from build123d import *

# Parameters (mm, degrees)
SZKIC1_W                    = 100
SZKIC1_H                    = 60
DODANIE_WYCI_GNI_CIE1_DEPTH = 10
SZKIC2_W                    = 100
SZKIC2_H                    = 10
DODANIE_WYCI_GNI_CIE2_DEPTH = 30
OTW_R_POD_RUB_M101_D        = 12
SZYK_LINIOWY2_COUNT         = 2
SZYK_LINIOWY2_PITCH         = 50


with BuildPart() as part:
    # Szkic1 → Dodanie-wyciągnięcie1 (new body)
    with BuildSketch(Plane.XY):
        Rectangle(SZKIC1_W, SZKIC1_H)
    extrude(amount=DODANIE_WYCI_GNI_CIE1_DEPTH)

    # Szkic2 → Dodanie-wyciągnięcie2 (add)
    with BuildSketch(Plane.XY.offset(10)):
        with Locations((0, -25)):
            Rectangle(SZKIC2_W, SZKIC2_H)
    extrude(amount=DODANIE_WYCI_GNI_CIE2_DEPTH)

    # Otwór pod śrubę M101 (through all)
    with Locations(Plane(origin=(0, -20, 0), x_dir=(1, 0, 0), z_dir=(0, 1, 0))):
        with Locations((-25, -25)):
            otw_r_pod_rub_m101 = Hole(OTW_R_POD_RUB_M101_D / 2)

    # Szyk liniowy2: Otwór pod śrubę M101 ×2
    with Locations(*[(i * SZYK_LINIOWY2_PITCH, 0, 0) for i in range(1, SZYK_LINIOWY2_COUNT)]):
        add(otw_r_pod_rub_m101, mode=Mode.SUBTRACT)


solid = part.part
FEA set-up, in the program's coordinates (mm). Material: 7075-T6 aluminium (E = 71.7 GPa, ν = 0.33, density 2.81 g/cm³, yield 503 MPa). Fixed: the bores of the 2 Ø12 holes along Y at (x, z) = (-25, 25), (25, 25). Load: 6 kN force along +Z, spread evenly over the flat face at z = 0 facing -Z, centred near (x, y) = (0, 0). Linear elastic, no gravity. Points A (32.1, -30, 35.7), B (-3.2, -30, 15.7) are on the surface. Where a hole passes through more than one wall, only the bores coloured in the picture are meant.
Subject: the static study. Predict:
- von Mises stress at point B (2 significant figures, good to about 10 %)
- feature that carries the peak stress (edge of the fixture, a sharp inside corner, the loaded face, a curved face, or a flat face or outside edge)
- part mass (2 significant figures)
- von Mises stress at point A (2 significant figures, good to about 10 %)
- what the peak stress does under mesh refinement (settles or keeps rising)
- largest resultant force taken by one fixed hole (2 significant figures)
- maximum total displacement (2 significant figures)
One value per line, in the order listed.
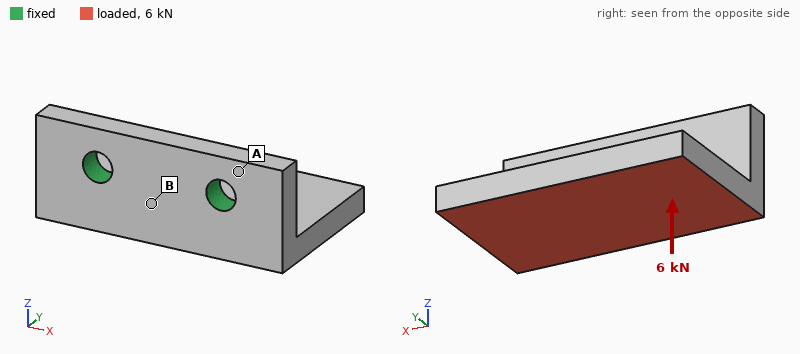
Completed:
56 MPa
edge of the fixture
250 g
21 MPa
keeps rising
3.0 kN
0.40 mm
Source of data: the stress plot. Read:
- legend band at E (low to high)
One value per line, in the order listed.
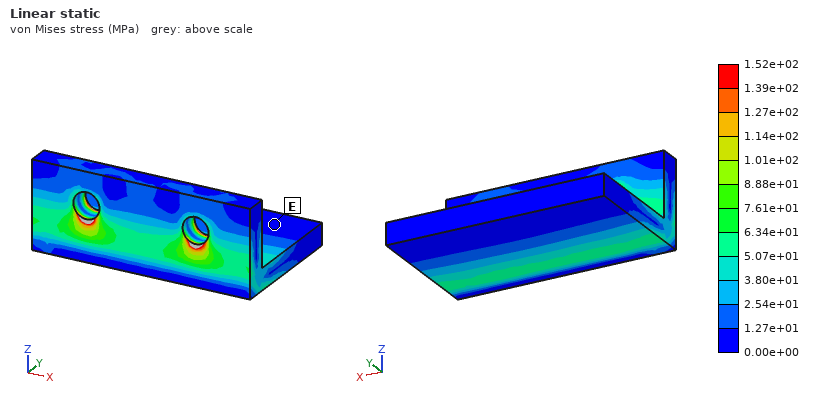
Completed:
0.00e+00 to 1.27e+01 MPa
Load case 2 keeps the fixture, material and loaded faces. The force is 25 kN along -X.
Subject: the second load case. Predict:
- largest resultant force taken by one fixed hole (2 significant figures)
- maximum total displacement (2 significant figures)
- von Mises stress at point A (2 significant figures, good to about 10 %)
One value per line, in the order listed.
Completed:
19 kN
0.20 mm
62 MPa
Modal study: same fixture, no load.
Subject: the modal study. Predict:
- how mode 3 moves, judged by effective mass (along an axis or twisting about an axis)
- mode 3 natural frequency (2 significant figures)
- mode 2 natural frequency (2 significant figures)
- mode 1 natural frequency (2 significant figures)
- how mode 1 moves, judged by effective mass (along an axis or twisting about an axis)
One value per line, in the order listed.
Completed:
along X
5000 Hz
3200 Hz
1800 Hz
along Z
